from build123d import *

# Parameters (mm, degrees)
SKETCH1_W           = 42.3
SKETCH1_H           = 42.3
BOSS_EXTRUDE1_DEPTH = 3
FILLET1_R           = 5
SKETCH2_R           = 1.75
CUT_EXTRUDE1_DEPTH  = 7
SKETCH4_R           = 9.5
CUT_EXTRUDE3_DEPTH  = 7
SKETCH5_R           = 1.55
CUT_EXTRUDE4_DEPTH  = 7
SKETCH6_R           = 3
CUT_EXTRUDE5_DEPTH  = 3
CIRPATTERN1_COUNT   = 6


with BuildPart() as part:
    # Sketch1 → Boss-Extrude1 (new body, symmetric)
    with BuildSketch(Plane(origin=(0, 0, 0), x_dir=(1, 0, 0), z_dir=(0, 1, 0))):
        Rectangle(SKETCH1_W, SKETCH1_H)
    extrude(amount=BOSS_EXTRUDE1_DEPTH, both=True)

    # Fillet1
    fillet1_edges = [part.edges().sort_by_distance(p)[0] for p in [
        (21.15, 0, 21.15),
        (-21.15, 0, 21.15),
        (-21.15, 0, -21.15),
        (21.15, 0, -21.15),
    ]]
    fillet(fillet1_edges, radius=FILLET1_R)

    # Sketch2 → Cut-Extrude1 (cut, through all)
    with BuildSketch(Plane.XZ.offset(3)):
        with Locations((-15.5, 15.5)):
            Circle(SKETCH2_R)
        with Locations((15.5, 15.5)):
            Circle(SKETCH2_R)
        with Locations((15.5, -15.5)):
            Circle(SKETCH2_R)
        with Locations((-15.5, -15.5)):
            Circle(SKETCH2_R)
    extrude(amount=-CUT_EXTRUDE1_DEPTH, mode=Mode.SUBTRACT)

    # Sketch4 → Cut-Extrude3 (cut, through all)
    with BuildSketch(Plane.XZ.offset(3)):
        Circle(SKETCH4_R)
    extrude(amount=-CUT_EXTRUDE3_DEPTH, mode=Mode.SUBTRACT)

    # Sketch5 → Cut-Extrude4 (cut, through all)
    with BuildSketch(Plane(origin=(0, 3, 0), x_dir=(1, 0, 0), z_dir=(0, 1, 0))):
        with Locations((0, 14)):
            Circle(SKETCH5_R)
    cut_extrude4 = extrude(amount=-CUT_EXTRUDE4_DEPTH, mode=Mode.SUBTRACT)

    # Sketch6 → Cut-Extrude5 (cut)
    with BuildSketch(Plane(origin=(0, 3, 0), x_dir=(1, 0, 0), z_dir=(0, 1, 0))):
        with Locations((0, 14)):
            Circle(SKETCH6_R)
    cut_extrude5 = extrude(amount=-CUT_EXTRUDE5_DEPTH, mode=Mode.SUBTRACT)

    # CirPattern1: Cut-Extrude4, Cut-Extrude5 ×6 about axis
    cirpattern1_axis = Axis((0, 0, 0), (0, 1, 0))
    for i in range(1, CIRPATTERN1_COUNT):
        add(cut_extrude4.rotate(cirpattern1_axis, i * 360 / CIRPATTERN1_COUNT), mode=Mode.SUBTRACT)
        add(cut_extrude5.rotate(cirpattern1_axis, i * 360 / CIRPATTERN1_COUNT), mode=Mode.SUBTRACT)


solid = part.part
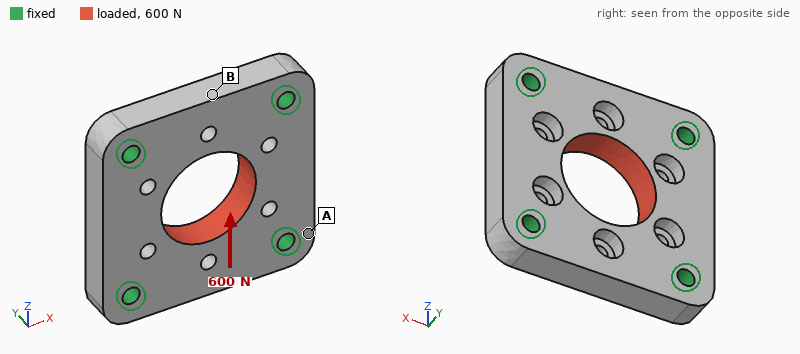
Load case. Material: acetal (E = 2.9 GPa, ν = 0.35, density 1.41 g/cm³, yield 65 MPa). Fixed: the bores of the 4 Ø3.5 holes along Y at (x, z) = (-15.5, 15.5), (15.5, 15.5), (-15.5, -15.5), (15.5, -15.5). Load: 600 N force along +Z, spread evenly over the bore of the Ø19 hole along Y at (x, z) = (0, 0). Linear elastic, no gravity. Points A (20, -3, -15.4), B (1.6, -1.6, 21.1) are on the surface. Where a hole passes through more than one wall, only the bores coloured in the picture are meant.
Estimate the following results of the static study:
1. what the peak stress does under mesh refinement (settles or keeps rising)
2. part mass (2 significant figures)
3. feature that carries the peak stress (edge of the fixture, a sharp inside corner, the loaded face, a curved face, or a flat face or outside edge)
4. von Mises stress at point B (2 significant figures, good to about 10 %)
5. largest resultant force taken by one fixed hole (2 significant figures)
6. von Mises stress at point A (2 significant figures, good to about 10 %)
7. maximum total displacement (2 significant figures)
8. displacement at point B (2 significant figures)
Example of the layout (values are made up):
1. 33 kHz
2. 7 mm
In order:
1. keeps rising
2. 11 g
3. edge of the fixture
4. 2.6 MPa
5. 160 N
6. 1.1 MPa
7. 29 µm
8. 19 µm
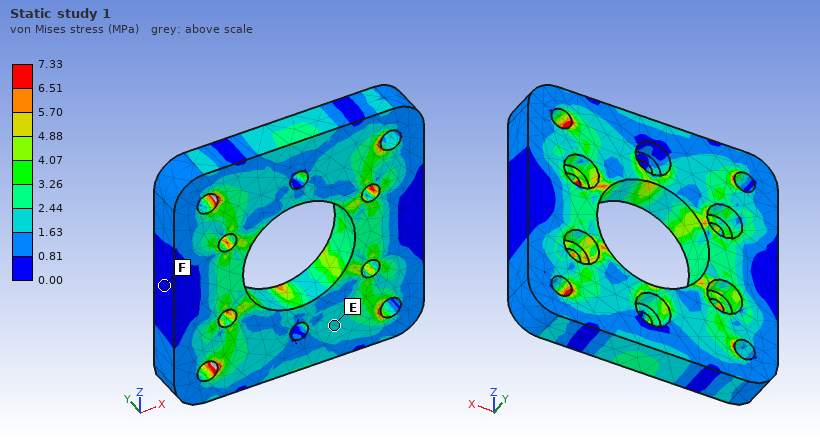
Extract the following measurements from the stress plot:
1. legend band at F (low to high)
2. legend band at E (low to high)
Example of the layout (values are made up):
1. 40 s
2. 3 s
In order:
1. 0.00 to 0.81 MPa
2. 1.63 to 2.44 MPa
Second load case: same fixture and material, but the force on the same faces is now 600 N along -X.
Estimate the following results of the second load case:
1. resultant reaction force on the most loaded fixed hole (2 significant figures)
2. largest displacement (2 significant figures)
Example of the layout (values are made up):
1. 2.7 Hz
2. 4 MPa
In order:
1. 160 N
2. 29 µm
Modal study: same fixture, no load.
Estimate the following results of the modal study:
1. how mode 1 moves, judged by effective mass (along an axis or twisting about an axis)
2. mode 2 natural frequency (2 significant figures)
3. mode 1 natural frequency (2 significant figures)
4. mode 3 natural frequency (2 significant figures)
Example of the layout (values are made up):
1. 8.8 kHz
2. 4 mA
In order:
1. along Y
2. 7900 Hz
3. 6800 Hz
4. 7900 Hz
